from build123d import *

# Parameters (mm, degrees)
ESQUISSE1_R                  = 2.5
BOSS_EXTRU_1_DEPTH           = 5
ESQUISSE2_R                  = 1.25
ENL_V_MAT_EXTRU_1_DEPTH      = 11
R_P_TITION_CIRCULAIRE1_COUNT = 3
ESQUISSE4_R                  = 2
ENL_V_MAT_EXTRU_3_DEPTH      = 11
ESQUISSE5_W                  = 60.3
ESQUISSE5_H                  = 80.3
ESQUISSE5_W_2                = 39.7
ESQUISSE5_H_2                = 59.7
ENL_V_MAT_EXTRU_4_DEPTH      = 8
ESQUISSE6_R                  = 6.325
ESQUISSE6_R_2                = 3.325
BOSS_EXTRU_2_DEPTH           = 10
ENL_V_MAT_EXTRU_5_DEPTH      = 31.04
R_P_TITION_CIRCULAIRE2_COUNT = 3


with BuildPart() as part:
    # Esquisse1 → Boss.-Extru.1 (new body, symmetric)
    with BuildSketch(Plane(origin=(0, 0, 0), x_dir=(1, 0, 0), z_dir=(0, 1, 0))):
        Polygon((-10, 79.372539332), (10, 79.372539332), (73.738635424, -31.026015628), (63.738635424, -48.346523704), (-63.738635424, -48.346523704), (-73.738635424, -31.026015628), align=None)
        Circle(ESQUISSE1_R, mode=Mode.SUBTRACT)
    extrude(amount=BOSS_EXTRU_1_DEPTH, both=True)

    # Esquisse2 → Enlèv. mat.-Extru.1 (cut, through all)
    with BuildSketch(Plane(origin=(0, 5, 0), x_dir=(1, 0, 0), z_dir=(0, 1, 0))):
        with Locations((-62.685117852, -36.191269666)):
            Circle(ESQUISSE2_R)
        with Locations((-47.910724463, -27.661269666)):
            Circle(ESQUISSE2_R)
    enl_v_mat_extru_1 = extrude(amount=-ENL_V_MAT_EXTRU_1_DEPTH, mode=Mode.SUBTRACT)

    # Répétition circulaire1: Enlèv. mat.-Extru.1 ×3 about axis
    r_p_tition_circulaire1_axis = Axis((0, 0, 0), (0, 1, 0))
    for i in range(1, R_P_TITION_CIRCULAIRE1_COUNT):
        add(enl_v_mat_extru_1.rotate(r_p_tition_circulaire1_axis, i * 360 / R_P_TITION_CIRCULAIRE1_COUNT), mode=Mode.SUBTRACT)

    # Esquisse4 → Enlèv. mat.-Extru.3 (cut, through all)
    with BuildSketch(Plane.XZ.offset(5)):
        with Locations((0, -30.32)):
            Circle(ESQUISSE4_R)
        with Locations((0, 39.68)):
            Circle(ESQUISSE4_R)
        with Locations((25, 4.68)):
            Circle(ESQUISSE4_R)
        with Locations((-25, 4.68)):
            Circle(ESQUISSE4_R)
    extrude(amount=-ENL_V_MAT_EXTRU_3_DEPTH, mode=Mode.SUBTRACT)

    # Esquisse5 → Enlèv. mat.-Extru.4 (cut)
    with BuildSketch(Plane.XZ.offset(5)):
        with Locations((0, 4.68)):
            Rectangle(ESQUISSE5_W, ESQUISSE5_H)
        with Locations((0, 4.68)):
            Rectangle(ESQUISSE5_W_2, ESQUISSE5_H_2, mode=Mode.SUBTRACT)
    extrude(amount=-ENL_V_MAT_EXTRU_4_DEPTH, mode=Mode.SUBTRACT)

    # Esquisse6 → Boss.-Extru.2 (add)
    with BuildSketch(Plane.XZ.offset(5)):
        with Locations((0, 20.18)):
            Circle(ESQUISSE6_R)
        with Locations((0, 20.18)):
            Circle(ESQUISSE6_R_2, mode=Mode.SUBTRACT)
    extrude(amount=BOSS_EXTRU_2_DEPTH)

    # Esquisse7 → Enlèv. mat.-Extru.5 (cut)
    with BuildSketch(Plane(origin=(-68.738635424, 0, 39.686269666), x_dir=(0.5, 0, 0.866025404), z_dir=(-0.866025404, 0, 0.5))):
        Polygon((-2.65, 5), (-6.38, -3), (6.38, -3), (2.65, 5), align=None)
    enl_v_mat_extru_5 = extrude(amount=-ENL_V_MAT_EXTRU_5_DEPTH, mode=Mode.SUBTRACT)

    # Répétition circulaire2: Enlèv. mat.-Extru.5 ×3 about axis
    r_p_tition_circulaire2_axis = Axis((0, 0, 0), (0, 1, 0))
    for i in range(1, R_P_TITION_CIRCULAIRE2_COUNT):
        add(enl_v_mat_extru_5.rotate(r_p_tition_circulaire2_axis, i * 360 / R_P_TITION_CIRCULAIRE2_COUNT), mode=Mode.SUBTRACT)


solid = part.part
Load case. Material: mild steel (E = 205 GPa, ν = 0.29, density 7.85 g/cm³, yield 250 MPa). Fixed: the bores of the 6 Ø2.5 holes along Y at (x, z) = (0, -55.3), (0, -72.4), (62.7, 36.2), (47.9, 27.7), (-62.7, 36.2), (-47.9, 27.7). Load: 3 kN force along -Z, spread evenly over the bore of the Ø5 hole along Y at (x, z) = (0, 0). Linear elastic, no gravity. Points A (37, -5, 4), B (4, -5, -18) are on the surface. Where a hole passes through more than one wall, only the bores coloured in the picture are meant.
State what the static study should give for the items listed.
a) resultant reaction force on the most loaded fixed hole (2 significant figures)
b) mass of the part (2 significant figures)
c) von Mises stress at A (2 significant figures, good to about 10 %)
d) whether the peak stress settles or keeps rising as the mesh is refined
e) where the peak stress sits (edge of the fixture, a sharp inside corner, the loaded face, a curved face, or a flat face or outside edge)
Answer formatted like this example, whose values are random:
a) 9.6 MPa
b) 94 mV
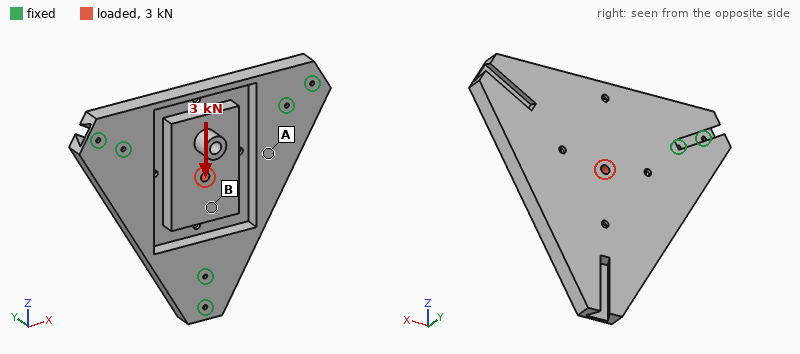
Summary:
a) 830 N
b) 710 g
c) 6.0 MPa
d) keeps rising
e) edge of the fixture
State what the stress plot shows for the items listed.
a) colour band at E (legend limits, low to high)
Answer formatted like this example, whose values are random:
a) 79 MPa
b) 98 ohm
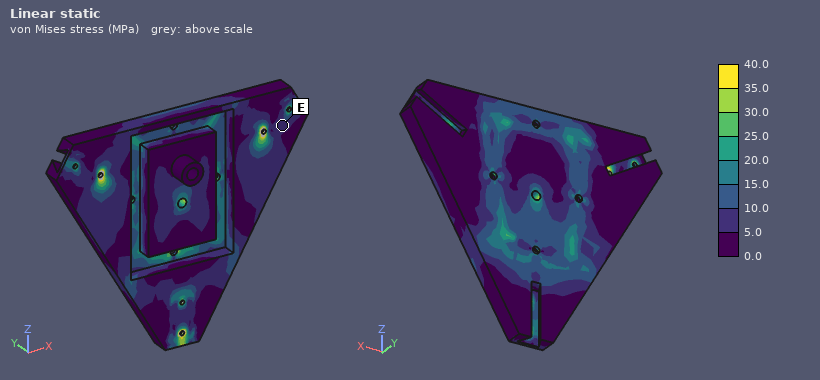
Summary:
a) 5.0 to 10.0 MPa
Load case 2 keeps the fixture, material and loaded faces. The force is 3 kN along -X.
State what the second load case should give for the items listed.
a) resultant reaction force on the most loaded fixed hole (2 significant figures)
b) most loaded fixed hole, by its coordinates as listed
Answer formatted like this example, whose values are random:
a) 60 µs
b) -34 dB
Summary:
a) 860 N
b) (0, -55.3)
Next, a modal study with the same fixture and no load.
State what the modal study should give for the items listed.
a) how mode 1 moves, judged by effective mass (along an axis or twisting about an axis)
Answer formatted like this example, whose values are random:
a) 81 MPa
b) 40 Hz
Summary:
a) along Y
